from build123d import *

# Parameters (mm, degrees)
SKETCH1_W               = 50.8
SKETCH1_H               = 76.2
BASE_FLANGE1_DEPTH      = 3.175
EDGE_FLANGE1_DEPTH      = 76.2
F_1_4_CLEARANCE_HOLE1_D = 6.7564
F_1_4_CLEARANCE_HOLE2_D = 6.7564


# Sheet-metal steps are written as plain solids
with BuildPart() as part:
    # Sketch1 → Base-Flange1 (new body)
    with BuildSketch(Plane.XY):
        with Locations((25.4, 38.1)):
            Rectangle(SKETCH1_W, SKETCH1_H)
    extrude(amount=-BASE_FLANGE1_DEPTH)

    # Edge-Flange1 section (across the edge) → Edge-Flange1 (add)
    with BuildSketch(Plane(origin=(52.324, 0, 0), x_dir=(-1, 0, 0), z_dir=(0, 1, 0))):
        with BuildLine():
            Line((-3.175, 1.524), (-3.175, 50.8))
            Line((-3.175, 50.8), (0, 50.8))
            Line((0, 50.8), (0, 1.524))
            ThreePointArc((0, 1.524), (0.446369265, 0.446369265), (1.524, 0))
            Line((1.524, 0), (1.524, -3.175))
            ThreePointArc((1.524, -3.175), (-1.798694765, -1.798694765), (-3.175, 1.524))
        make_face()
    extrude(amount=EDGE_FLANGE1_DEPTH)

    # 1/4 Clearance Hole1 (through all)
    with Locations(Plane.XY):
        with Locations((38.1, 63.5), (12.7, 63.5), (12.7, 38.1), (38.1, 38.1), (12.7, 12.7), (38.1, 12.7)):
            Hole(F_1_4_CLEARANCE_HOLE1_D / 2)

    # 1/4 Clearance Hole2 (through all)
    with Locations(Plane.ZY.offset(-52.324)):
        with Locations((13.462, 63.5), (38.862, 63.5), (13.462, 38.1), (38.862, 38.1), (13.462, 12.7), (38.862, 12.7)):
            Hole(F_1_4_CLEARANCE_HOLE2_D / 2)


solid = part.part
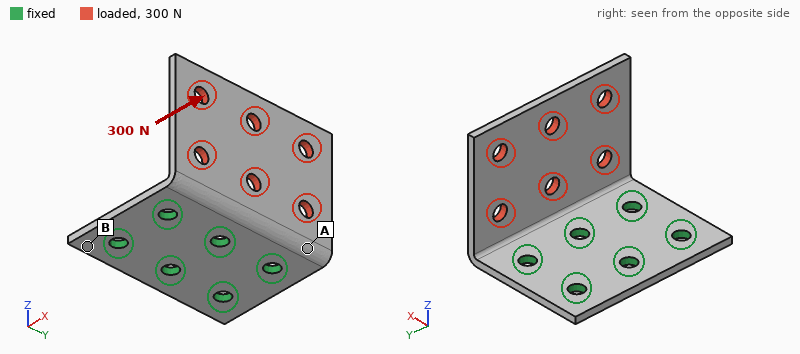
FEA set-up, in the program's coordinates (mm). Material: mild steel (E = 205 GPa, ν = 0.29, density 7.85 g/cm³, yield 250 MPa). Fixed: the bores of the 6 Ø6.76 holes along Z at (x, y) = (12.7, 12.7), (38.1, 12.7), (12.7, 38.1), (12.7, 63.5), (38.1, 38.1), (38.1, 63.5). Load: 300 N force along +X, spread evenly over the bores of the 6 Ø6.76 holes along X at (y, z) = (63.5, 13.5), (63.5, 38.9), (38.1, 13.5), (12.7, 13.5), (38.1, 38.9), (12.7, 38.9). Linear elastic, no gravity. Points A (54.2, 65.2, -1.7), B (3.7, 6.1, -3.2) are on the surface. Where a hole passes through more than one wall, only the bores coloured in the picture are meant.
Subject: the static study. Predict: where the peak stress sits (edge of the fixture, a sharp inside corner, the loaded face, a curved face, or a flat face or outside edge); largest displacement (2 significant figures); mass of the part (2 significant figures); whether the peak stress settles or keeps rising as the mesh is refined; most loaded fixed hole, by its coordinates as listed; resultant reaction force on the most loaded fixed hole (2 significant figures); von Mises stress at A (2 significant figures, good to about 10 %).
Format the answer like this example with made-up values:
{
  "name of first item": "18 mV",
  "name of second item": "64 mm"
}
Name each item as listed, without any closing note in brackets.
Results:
{
  "where the peak stress sits": "edge of the fixture",
  "largest displacement": "0.27 mm",
  "mass of the part": "190 g",
  "whether the peak stress settles or keeps rising as the mesh is refined": "keeps rising",
  "most loaded fixed hole, by its coordinates as listed": "(38.1, 38.1)",
  "resultant reaction force on the most loaded fixed hole": "100 N",
  "von Mises stress at A": "39 MPa"
}
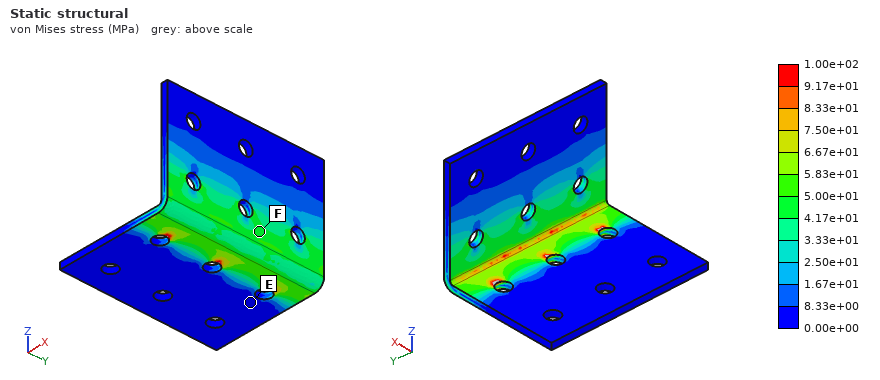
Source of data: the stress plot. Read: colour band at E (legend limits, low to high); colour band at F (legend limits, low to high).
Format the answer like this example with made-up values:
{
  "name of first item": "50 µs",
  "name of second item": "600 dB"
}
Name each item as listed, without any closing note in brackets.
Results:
{
  "colour band at E": "0.00e+00 to 8.33e+00 MPa",
  "colour band at F": "4.17e+01 to 5.00e+01 MPa"
}
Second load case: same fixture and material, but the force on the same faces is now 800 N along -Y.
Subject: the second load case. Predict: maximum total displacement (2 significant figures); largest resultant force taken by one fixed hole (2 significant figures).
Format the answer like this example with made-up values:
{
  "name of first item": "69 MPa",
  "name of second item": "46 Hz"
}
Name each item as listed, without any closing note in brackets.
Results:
{
  "maximum total displacement": "63 µm",
  "largest resultant force taken by one fixed hole": "520 N"
}
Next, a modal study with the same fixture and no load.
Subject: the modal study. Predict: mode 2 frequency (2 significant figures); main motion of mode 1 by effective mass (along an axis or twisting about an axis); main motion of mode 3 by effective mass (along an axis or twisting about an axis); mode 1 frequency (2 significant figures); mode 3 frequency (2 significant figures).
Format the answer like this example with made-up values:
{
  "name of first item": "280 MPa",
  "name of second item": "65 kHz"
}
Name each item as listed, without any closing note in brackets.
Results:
{
  "mode 2 frequency": "1500 Hz",
  "main motion of mode 1 by effective mass": "along X",
  "main motion of mode 3 by effective mass": "along Y",
  "mode 1 frequency": "690 Hz",
  "mode 3 frequency": "2700 Hz"
}
